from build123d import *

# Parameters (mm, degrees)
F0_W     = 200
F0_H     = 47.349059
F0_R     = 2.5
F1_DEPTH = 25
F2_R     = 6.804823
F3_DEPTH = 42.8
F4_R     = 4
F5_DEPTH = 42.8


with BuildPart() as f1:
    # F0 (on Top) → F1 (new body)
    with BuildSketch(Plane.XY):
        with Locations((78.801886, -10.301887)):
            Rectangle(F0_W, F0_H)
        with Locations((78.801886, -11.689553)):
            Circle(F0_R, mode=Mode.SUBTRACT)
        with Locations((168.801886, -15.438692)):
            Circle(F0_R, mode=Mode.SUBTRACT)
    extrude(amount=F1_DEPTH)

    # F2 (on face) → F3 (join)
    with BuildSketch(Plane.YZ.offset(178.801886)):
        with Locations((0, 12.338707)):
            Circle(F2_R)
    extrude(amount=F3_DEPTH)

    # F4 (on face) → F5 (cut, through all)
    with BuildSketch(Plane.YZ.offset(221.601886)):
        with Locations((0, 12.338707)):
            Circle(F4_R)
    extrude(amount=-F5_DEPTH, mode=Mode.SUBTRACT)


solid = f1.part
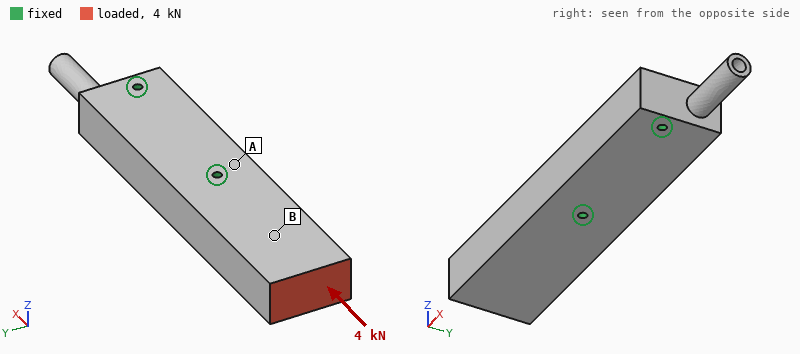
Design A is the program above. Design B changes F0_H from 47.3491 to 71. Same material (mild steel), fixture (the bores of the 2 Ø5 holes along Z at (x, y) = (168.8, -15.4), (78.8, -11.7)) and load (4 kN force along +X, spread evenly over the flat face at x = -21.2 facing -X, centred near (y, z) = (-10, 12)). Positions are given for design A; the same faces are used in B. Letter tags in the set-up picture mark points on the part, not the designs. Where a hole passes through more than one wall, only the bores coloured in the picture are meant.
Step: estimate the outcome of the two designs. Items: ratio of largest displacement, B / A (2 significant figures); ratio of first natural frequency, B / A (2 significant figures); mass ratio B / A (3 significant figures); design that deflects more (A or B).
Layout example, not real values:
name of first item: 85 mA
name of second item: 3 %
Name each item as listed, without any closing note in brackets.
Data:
ratio of largest displacement, B / A: 0.73
ratio of first natural frequency, B / A: 0.95
mass ratio B / A: 1.49
design that deflects more: A
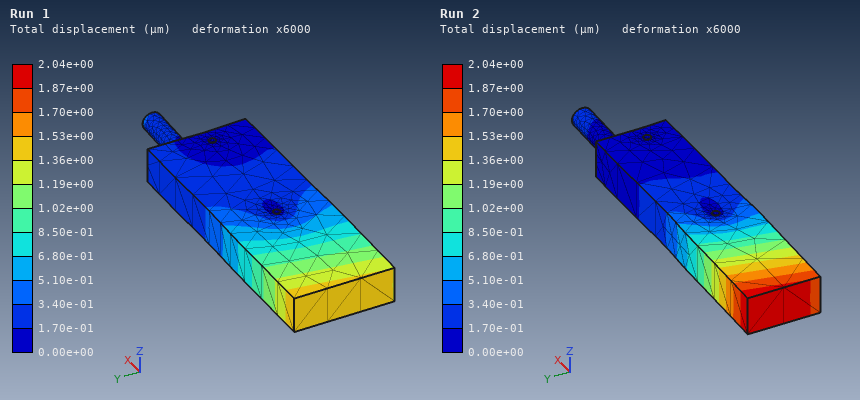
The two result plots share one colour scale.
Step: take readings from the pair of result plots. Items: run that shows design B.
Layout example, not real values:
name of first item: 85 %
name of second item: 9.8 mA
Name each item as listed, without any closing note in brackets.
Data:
run that shows design B: Run 1
